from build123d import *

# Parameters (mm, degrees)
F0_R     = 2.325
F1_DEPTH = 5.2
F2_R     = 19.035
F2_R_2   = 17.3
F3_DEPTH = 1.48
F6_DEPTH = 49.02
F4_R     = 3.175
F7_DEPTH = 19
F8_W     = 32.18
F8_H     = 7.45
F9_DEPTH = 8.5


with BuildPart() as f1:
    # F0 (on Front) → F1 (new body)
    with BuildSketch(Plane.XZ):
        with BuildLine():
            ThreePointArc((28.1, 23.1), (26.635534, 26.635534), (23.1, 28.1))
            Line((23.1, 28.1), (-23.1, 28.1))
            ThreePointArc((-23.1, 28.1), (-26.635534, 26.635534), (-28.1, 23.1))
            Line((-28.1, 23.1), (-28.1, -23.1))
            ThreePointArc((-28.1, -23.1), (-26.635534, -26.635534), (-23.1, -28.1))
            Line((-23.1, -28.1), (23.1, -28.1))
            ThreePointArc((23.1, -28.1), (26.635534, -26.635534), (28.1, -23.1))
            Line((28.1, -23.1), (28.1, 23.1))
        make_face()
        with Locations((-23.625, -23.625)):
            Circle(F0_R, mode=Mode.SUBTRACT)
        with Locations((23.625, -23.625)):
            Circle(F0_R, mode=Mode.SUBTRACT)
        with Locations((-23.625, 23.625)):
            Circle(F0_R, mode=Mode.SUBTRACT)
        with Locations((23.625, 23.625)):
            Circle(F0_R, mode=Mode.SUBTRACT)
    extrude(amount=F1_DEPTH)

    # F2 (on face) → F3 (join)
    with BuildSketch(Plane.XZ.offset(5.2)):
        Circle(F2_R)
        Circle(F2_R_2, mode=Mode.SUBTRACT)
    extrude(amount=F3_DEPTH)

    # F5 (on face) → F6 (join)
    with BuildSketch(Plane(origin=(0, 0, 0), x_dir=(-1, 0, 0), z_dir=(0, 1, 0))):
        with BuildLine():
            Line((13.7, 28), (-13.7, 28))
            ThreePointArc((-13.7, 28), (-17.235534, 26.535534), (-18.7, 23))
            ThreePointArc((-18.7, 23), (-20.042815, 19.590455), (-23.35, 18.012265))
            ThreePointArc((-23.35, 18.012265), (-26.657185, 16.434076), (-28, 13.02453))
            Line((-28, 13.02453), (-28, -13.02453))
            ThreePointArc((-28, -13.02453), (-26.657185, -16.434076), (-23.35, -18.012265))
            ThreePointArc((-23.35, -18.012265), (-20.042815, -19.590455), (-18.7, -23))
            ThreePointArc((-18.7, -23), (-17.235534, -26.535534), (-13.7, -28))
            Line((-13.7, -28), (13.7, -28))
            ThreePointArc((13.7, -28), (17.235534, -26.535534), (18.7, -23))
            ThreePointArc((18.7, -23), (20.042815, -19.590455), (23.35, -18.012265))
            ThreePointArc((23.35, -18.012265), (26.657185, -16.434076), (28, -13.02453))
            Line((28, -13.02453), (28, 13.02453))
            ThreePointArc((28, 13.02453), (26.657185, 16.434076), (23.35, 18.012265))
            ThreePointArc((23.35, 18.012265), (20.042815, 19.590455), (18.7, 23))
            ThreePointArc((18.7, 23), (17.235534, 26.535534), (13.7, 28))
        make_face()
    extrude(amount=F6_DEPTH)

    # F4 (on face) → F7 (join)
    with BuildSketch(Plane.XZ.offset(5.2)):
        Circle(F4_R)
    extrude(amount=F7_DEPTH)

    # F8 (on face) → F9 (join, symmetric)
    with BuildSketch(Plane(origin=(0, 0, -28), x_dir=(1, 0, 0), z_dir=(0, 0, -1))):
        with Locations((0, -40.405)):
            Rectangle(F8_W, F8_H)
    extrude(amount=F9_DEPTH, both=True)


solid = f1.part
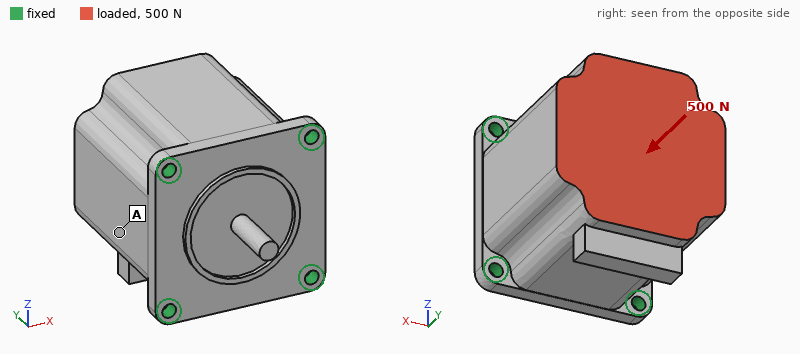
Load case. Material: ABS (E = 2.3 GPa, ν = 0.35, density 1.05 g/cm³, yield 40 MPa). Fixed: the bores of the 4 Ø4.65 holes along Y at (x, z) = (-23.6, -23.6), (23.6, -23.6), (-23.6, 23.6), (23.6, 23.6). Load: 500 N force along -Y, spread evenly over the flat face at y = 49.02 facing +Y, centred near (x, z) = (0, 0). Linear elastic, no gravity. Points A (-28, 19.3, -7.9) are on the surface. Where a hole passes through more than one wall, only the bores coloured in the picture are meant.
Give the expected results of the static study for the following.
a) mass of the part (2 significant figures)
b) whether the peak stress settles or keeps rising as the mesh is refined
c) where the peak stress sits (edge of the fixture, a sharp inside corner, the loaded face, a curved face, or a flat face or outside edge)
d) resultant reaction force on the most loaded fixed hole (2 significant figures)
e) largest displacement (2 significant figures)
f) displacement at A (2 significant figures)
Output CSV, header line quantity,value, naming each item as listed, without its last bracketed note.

quantity,value
mass of the part,160 g
whether the peak stress settles or keeps rising as the mesh is refined,keeps rising
where the peak stress sits,edge of the fixture
resultant reaction force on the most loaded fixed hole,130 N
largest displacement,23 µm
displacement at A,21 µm
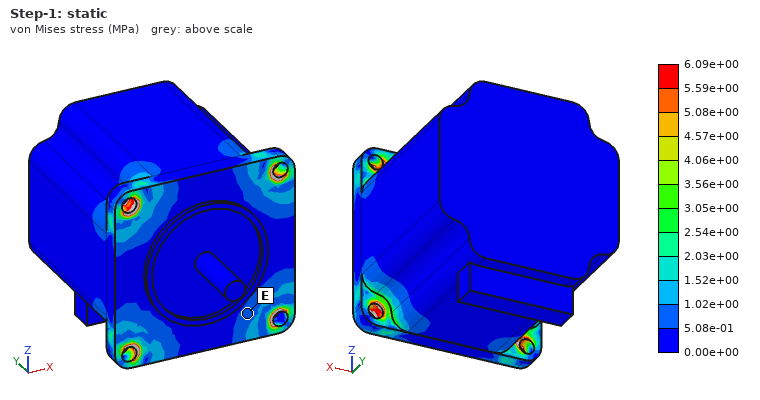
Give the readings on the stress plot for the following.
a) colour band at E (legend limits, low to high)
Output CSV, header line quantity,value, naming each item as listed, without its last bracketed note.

quantity,value
colour band at E,5.08e-01 to 1.02e+00 MPa
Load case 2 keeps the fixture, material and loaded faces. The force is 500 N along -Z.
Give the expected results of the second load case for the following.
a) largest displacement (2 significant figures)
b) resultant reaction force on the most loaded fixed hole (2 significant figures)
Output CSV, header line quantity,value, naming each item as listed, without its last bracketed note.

quantity,value
largest displacement,0.15 mm
resultant reaction force on the most loaded fixed hole,330 N
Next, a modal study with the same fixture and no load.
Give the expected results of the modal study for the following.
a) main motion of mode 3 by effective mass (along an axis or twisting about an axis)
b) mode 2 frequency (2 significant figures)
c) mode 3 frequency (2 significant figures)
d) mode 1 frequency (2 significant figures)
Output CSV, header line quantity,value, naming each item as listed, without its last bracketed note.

quantity,value
main motion of mode 3 by effective mass,along Y
mode 2 frequency,1200 Hz
mode 3 frequency,2000 Hz
mode 1 frequency,1200 Hz
